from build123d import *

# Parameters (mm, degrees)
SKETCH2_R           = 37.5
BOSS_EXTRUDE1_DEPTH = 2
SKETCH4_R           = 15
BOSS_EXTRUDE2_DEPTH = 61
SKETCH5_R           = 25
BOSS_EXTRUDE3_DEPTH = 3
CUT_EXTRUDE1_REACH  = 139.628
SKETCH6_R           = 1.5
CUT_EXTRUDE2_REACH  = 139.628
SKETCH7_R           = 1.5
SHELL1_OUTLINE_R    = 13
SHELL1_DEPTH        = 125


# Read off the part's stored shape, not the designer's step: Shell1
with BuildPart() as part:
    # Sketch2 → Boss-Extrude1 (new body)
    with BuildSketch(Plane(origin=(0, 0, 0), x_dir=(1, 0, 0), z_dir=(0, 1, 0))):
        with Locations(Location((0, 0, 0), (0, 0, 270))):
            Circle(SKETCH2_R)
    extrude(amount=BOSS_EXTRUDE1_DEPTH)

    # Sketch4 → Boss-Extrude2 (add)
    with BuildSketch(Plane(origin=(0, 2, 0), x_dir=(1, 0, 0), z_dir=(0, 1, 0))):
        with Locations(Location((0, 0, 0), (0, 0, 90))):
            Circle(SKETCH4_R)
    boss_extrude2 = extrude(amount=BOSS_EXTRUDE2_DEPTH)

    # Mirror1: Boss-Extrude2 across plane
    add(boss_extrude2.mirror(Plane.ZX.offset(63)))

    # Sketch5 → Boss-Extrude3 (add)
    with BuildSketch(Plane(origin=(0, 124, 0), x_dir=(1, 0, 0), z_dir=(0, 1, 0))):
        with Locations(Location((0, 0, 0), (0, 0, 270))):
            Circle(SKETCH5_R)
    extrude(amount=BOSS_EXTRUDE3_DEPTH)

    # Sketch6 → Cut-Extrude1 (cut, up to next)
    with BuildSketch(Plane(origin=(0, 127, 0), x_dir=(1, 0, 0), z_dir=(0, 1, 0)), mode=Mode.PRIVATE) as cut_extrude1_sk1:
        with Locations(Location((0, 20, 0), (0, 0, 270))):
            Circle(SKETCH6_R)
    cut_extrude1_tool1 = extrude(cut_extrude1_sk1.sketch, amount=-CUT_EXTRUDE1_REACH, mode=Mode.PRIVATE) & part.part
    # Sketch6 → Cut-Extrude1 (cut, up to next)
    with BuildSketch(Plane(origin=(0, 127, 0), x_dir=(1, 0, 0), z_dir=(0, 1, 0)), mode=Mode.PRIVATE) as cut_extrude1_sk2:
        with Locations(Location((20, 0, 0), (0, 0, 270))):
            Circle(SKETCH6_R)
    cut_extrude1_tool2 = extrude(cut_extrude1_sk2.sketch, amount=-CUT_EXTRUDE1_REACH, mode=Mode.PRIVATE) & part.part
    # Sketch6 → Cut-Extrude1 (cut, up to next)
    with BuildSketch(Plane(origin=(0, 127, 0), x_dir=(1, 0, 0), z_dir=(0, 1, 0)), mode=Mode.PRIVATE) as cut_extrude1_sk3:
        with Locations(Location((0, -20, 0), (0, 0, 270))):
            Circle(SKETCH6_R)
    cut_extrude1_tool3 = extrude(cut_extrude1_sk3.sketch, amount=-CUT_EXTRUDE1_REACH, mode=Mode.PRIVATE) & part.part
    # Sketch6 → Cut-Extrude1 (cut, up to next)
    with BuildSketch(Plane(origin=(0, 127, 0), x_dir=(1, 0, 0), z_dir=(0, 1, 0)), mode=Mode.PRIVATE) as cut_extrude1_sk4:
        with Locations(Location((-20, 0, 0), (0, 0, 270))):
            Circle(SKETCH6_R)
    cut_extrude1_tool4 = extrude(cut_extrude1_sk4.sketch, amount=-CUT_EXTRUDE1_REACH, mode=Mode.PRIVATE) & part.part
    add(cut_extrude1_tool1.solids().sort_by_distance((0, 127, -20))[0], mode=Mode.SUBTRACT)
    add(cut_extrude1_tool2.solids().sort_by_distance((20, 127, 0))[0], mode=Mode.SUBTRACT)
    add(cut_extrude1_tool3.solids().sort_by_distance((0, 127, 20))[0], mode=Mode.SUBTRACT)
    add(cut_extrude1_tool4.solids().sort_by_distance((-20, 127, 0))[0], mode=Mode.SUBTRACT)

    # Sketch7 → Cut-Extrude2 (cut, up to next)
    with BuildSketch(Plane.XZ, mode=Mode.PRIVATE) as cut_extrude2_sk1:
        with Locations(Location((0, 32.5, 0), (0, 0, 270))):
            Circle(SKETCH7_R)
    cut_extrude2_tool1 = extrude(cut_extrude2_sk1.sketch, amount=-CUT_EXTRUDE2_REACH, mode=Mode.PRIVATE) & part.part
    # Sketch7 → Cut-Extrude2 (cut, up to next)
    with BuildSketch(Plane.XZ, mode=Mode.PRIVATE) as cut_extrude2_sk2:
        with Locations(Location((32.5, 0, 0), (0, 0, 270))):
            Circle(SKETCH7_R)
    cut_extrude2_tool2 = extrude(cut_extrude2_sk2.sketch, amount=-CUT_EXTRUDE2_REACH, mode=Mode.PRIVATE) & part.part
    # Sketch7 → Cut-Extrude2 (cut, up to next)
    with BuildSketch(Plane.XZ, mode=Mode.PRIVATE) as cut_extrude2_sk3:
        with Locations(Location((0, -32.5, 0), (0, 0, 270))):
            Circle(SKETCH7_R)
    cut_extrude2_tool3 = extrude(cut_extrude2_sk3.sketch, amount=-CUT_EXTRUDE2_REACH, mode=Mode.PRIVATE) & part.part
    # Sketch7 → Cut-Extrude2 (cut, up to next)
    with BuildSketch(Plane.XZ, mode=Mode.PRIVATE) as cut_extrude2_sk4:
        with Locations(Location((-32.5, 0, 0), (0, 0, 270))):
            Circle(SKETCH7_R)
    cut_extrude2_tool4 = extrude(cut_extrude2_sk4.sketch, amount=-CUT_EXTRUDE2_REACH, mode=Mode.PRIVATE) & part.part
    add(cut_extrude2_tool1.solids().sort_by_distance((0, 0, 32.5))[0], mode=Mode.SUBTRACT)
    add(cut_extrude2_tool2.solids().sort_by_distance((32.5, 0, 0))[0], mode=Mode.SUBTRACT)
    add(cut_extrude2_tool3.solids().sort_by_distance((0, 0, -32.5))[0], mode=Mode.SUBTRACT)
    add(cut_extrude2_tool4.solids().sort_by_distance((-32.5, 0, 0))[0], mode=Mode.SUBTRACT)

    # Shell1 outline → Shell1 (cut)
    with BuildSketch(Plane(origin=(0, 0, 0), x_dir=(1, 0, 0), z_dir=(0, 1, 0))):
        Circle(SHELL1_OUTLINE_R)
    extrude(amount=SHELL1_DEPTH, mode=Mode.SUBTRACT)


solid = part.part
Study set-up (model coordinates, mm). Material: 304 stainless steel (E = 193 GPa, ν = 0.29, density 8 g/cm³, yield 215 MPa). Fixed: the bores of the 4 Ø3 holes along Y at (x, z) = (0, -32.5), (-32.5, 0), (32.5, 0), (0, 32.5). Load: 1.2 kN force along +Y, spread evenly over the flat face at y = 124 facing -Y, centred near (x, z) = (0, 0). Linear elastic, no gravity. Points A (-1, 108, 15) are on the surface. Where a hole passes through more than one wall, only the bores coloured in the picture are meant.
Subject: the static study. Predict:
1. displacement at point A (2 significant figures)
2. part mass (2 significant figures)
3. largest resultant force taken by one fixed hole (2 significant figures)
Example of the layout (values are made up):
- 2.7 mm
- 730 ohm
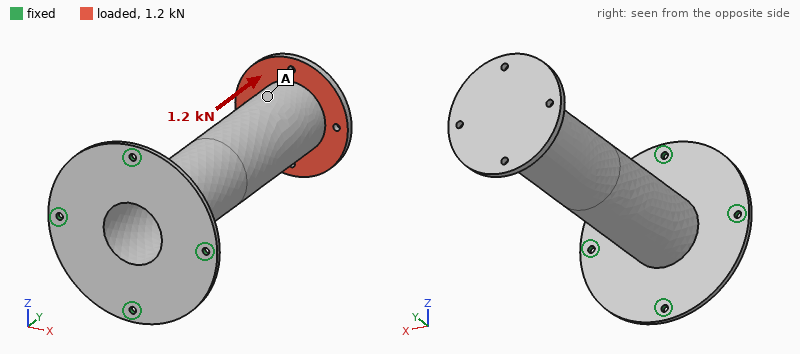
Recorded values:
- 68 µm
- 280 g
- 360 N
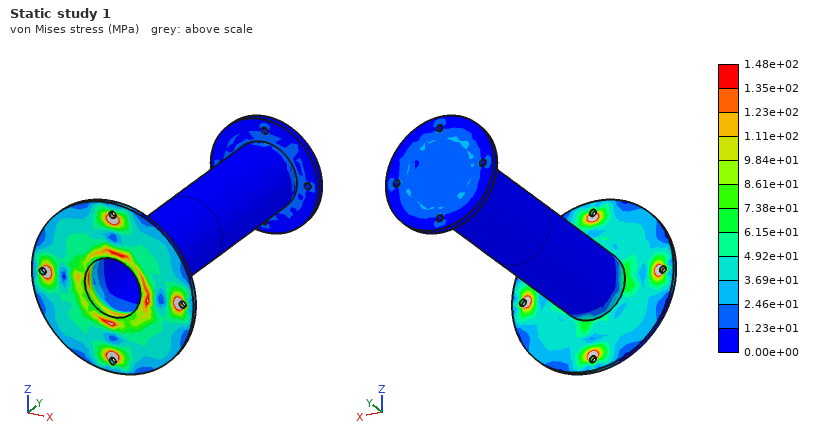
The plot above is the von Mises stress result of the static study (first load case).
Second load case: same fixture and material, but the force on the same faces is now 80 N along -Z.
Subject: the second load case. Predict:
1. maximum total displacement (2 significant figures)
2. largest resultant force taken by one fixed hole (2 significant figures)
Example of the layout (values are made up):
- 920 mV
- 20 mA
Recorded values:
- 0.22 mm
- 180 N
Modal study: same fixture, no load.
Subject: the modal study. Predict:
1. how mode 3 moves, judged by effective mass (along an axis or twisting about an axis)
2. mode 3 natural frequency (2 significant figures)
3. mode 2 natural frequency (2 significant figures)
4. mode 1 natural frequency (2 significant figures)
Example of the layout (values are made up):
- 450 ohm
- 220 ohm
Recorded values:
- along Y
- 1400 Hz
- 310 Hz
- 310 Hz
